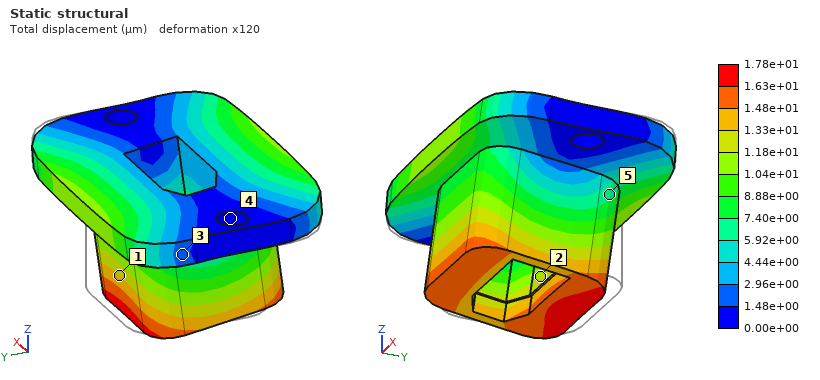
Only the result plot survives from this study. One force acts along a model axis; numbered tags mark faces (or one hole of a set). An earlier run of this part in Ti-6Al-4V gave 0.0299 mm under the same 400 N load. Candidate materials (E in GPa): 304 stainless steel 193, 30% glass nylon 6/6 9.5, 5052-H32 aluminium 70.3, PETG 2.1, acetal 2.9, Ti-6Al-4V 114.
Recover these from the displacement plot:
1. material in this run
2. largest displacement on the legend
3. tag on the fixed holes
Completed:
304 stainless steel
1.78e+01 µm
4
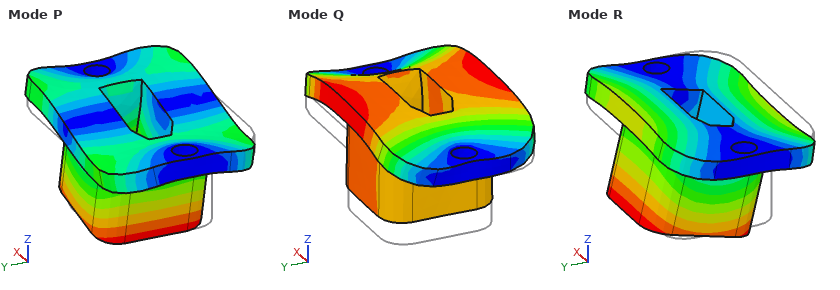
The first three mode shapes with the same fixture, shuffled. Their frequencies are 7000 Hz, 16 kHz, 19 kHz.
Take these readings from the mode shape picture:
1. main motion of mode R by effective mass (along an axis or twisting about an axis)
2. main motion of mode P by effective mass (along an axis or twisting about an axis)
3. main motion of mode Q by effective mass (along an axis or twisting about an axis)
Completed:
along Y
along X
along Z
